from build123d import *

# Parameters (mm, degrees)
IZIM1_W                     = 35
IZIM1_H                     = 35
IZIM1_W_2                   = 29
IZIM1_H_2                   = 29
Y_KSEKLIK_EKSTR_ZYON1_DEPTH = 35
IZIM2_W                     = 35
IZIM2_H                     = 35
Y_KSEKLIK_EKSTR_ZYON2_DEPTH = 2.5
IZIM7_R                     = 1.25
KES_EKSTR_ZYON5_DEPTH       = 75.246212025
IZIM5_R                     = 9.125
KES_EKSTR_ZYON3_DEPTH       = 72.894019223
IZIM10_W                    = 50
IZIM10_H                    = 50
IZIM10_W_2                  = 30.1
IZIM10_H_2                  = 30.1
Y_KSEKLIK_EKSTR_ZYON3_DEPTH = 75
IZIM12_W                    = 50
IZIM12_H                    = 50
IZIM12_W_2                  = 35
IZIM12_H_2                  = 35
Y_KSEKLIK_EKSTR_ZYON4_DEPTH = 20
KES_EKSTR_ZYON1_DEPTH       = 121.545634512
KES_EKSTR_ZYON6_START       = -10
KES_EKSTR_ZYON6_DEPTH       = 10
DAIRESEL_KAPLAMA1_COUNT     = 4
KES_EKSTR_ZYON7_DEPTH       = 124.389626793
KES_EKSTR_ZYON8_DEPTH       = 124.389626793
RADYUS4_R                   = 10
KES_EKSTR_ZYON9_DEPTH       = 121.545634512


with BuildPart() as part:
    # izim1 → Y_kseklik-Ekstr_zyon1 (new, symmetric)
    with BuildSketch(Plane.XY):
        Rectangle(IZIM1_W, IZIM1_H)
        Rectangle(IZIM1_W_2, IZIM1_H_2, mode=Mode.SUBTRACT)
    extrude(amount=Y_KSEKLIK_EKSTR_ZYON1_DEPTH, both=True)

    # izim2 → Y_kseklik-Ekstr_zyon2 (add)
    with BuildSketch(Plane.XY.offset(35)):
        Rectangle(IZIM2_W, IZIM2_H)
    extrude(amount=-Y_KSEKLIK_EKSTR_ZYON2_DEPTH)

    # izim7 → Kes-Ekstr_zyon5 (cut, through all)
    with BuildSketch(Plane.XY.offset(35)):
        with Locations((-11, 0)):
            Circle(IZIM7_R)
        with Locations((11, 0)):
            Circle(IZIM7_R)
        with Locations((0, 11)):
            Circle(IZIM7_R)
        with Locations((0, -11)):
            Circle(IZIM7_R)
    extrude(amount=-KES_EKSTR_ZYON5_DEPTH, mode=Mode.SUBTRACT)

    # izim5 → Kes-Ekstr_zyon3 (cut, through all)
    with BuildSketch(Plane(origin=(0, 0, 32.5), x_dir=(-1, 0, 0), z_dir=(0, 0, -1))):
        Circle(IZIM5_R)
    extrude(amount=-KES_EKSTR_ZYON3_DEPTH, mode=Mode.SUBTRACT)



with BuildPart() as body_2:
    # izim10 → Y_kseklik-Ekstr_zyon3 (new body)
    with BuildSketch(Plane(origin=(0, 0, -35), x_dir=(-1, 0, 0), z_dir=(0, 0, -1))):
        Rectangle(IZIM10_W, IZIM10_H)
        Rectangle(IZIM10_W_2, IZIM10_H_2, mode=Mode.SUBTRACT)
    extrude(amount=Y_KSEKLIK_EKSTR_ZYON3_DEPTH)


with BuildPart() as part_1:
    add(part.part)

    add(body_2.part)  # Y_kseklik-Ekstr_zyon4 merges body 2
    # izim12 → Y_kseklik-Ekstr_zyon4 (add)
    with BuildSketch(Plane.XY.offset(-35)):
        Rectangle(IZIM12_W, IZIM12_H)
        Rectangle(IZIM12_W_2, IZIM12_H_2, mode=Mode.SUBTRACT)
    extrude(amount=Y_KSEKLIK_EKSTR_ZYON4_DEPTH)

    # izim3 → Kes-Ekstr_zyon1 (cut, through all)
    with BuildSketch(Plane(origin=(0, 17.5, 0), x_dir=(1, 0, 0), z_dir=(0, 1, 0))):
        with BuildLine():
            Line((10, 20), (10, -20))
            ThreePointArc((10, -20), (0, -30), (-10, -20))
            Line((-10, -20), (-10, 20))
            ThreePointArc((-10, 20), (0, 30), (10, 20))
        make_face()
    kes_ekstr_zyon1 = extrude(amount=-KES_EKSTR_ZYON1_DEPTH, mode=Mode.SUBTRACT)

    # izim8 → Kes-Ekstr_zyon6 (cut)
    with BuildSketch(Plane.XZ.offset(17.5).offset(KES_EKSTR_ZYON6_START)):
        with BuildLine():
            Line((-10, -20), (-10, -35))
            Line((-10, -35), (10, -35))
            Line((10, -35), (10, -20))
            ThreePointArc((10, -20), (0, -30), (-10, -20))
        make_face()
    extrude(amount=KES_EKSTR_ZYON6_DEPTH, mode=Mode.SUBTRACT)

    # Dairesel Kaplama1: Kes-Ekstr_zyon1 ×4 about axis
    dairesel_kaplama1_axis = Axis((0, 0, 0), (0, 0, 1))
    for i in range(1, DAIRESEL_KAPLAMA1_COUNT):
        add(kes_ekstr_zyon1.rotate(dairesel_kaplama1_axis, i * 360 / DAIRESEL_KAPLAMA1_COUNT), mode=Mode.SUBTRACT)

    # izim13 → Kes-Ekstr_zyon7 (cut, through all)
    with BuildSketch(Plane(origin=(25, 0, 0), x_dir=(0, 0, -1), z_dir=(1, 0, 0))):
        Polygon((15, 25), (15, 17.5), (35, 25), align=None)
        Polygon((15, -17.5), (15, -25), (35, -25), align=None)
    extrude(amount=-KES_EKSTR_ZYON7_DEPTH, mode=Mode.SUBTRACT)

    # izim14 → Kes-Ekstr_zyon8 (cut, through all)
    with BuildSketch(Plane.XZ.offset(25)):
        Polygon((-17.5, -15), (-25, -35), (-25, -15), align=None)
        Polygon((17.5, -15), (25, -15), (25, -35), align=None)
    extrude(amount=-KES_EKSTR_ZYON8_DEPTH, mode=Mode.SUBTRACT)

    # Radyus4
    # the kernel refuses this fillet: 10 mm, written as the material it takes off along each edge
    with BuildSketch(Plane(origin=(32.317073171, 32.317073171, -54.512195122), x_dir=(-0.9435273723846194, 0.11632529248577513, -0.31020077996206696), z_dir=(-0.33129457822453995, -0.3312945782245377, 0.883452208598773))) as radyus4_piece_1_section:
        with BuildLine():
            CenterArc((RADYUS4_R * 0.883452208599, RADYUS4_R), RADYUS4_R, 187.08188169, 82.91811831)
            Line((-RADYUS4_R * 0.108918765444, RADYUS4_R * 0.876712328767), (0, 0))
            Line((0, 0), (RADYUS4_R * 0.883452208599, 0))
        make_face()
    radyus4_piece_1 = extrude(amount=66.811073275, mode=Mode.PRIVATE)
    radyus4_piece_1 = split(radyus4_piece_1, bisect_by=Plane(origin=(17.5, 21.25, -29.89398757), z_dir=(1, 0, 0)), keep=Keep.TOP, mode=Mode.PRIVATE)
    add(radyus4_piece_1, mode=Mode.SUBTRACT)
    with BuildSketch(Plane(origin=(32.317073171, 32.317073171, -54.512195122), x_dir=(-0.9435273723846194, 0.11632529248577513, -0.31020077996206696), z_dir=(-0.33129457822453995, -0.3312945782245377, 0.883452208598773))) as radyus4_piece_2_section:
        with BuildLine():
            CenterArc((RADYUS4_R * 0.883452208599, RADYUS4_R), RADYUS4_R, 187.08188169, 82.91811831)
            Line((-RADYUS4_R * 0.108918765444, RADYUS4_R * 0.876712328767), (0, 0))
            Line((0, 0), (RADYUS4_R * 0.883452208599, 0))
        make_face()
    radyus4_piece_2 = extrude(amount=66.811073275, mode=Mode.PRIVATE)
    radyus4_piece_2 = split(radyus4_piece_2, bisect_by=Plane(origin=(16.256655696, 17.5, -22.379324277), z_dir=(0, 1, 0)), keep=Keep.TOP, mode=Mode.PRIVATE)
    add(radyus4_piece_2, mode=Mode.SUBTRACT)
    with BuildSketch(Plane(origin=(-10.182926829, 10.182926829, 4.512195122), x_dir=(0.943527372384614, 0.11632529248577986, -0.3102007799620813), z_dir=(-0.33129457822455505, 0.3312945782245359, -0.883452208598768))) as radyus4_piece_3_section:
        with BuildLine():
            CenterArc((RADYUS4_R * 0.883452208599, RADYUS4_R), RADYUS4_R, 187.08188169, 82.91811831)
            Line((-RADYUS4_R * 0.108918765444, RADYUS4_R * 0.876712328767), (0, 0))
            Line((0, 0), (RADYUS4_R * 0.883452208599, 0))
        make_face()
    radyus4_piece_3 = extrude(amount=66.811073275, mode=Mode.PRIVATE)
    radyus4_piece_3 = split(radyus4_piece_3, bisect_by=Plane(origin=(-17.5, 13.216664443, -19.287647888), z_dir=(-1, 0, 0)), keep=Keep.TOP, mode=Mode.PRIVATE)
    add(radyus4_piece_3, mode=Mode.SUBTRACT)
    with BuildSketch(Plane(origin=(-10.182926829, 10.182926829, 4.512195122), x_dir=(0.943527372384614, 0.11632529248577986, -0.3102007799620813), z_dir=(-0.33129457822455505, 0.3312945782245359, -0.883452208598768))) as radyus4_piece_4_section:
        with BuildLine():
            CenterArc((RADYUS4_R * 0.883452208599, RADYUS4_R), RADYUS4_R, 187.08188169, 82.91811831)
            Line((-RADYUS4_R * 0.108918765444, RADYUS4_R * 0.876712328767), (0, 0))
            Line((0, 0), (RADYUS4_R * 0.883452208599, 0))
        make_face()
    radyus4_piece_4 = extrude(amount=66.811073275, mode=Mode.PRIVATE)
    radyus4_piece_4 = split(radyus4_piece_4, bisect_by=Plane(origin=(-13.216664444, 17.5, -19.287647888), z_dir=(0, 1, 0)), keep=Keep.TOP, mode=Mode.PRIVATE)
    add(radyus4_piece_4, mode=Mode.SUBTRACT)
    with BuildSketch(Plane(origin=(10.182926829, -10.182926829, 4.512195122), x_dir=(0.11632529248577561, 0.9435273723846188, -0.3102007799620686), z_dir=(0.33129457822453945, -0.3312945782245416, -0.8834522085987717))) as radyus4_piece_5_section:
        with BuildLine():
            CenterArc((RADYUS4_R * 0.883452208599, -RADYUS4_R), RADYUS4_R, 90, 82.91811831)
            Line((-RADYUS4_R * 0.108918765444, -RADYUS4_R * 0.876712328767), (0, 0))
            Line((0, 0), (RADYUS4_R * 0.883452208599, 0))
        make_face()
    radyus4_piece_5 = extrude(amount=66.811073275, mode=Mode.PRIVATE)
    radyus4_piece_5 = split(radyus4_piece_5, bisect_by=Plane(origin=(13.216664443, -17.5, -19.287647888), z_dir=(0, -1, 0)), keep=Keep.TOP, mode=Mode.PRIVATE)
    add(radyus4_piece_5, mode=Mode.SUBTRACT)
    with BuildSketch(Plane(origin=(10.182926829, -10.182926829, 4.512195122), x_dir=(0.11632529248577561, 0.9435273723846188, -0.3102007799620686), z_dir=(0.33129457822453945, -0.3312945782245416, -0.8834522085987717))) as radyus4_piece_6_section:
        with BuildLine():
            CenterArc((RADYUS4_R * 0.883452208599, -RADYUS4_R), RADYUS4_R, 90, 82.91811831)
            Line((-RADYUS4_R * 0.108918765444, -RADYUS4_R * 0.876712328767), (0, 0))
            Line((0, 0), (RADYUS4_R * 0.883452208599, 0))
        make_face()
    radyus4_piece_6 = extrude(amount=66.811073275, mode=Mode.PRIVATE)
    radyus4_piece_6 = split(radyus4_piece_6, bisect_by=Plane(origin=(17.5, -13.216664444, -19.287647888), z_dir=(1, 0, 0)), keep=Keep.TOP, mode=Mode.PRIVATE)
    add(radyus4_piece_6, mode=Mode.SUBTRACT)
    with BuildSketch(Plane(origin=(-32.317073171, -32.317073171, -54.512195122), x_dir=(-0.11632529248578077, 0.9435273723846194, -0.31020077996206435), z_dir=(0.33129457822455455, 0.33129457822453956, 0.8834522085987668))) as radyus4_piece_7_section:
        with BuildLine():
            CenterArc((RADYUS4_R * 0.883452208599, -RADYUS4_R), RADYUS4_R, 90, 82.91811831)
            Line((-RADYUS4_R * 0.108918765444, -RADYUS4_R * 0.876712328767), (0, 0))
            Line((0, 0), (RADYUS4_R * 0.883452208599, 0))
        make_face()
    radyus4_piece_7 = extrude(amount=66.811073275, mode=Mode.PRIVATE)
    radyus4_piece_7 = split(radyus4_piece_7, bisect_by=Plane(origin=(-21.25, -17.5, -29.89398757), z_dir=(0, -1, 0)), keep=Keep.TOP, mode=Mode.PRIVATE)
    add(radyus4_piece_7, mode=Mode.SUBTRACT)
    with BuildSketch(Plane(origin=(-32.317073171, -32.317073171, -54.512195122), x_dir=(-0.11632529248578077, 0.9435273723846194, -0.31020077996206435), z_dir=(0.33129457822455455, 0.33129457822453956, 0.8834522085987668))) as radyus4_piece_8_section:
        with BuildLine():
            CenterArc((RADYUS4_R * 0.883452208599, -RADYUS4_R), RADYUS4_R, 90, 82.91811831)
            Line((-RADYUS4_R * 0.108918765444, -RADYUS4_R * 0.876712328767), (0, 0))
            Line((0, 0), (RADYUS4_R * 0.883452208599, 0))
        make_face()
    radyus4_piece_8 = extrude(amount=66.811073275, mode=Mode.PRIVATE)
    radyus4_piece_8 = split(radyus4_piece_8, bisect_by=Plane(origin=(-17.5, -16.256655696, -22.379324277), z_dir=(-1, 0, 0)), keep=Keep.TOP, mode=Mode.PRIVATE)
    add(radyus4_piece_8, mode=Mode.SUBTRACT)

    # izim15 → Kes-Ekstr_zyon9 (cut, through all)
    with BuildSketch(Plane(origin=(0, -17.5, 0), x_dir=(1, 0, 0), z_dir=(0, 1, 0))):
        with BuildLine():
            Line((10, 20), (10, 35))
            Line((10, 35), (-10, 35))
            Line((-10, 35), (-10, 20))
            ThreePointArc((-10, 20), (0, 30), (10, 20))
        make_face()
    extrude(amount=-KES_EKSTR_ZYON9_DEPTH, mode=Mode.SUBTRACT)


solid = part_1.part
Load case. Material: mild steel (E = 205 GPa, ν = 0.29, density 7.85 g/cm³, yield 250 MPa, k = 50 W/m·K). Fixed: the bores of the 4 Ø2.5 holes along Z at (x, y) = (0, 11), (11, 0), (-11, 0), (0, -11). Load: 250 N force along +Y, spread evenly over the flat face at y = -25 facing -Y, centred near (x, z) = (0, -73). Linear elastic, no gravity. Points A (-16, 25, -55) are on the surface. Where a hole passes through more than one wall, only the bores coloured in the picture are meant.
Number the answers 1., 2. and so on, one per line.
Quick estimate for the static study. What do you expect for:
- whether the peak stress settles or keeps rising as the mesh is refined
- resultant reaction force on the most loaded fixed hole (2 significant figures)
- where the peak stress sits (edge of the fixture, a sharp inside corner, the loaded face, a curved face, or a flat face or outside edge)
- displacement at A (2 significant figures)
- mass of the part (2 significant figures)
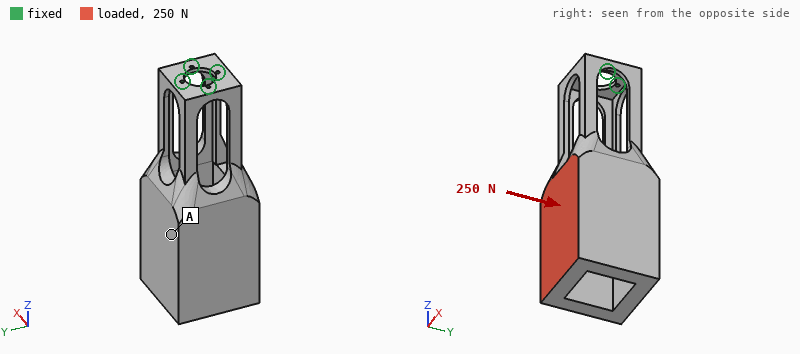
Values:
1. keeps rising
2. 860 N
3. edge of the fixture
4. 0.14 mm
5. 1.1 kg
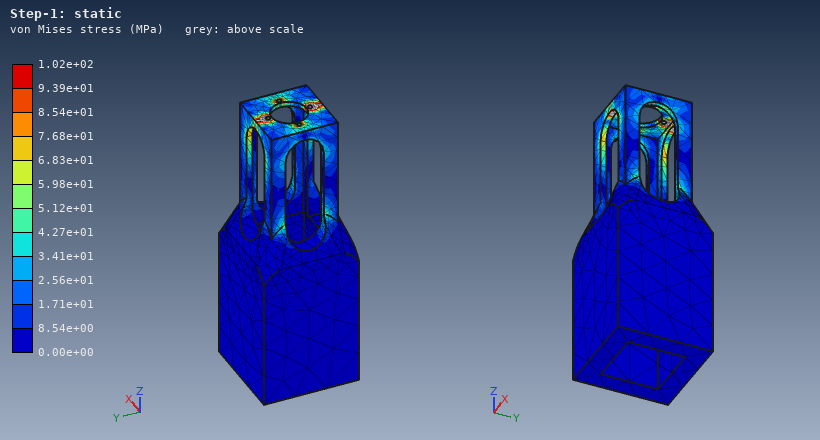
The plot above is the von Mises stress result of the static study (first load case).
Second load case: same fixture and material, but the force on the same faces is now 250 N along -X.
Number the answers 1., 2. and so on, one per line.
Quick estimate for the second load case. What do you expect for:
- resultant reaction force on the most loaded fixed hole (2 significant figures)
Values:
1. 870 N
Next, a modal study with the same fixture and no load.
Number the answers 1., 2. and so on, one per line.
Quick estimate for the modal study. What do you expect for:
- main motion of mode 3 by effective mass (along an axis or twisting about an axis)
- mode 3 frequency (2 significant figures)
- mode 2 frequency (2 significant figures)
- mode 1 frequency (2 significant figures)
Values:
1. twisting about Z
2. 550 Hz
3. 190 Hz
4. 190 Hz
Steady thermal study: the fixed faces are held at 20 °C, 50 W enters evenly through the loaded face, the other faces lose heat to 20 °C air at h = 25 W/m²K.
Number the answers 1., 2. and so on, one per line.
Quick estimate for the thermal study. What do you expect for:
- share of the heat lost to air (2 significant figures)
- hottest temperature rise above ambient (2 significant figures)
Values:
1. 90 %
2. 77 K
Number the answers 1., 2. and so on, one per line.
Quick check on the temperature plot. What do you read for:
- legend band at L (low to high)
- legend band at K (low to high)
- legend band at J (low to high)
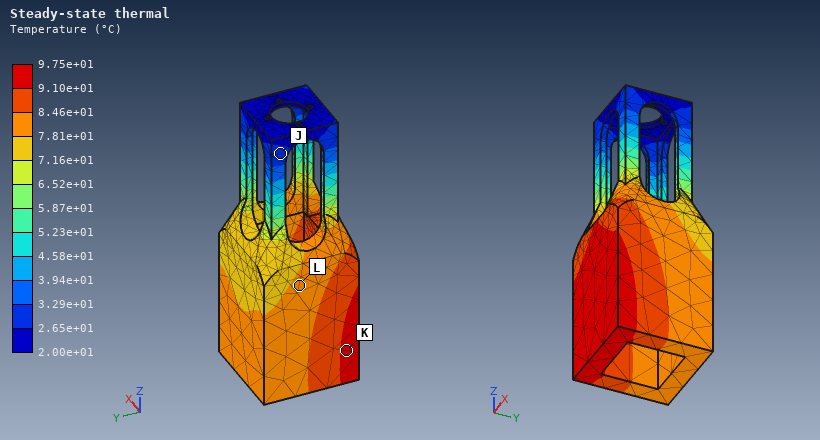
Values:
1. 7.81e+01 to 8.46e+01 °C
2. 9.10e+01 to 9.75e+01 °C
3. 2.65e+01 to 3.29e+01 °C
